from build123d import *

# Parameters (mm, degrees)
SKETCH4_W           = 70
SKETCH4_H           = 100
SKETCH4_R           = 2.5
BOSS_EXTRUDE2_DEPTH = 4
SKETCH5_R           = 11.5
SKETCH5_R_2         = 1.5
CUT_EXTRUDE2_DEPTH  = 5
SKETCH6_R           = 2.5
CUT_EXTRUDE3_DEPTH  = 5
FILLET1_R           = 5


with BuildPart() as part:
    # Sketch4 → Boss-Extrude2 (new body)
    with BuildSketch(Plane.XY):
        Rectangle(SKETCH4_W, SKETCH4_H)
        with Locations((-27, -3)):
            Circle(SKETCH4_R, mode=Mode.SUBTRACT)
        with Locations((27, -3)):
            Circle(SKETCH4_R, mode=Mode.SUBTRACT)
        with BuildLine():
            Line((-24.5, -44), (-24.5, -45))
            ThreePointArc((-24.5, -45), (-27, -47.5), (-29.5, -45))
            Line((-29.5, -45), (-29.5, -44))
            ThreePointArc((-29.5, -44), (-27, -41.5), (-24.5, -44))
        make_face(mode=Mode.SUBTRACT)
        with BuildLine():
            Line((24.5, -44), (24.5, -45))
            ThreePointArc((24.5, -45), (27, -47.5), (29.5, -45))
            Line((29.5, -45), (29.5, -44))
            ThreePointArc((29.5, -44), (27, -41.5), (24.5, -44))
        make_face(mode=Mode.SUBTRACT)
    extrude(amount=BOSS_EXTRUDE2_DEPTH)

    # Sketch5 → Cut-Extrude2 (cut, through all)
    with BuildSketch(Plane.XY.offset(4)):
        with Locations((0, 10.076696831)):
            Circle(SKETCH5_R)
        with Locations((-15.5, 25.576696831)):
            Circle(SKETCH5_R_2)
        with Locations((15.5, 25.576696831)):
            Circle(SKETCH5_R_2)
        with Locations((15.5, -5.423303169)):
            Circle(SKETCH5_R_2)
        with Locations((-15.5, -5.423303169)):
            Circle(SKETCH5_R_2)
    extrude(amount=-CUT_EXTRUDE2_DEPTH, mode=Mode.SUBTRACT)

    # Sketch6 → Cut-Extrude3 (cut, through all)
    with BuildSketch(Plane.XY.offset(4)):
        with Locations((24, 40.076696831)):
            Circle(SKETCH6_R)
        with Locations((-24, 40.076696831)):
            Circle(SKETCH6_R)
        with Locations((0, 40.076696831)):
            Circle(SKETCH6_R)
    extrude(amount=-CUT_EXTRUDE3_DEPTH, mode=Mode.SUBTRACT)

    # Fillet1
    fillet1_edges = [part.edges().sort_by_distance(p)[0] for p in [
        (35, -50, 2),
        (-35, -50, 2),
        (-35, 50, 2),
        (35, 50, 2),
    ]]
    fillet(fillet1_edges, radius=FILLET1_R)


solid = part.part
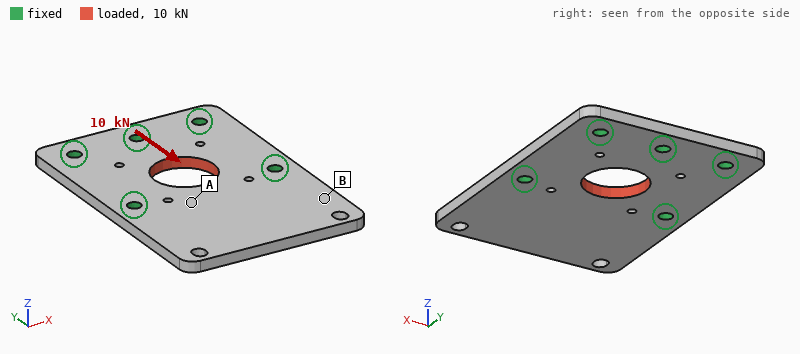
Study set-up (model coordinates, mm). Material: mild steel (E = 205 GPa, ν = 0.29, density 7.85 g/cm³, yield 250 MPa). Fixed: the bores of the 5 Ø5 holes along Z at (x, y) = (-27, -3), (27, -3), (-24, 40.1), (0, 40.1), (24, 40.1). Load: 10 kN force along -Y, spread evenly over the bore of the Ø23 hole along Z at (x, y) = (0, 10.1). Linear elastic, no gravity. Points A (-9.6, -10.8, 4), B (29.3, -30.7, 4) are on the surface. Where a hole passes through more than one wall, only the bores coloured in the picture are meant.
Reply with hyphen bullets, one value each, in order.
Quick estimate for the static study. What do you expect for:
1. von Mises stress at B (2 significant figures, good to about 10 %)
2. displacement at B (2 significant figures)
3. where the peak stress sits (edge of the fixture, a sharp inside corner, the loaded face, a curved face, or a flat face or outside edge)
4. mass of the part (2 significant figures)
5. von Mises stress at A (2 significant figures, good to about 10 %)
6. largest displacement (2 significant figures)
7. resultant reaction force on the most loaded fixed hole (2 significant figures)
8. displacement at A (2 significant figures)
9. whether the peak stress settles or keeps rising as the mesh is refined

- 7.5 MPa
- 1.9 µm
- edge of the fixture
- 200 g
- 24 MPa
- 6.3 µm
- 2.5 kN
- 4.1 µm
- keeps rising
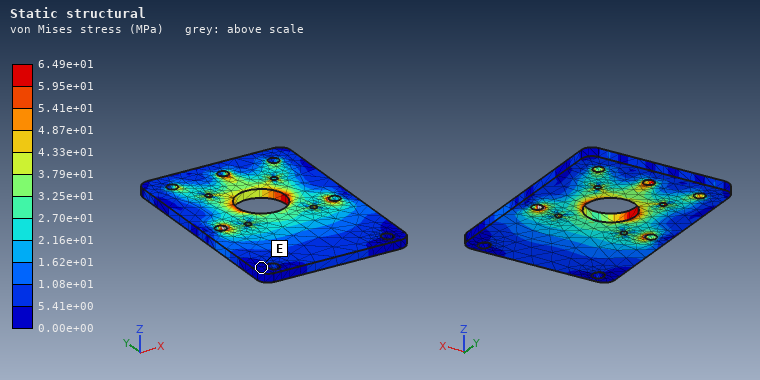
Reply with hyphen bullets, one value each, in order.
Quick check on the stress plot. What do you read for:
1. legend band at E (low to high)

- 0.00e+00 to 5.41e+00 MPa
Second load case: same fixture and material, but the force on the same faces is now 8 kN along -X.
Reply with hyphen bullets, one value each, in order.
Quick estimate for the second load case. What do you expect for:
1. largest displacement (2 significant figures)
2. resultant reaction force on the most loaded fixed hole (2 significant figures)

- 4.4 µm
- 2.5 kN
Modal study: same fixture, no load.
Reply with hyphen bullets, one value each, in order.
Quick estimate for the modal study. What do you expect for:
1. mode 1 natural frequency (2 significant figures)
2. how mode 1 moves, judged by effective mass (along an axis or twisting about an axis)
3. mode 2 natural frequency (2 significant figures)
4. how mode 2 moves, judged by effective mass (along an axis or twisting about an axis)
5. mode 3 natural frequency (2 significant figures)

- 1400 Hz
- along Z
- 2900 Hz
- twisting about Y
- 5900 Hz
